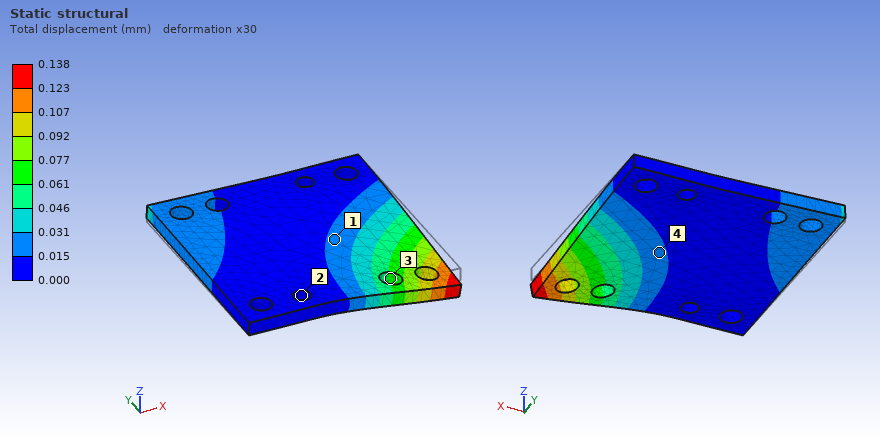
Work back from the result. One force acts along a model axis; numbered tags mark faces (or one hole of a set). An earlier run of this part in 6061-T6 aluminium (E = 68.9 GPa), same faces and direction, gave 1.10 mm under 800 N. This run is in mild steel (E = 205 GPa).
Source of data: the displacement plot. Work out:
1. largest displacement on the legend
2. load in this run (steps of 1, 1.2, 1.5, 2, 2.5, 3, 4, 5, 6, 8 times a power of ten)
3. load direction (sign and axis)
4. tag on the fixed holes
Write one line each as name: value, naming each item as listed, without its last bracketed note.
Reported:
largest displacement on the legend: 0.138 mm
load in this run: 300 N
load direction: -Z
tag on the fixed holes: 2
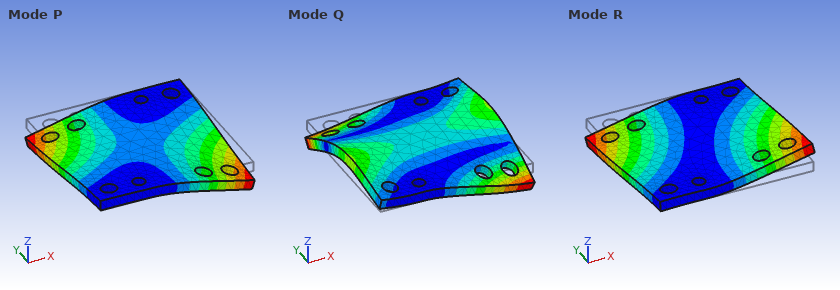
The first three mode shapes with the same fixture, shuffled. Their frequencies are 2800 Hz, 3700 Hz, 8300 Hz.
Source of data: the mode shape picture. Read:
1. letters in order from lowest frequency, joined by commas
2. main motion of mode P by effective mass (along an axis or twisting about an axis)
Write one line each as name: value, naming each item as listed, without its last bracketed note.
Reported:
letters in order from lowest frequency, joined by commas: R, P, Q
main motion of mode P by effective mass: along Z
